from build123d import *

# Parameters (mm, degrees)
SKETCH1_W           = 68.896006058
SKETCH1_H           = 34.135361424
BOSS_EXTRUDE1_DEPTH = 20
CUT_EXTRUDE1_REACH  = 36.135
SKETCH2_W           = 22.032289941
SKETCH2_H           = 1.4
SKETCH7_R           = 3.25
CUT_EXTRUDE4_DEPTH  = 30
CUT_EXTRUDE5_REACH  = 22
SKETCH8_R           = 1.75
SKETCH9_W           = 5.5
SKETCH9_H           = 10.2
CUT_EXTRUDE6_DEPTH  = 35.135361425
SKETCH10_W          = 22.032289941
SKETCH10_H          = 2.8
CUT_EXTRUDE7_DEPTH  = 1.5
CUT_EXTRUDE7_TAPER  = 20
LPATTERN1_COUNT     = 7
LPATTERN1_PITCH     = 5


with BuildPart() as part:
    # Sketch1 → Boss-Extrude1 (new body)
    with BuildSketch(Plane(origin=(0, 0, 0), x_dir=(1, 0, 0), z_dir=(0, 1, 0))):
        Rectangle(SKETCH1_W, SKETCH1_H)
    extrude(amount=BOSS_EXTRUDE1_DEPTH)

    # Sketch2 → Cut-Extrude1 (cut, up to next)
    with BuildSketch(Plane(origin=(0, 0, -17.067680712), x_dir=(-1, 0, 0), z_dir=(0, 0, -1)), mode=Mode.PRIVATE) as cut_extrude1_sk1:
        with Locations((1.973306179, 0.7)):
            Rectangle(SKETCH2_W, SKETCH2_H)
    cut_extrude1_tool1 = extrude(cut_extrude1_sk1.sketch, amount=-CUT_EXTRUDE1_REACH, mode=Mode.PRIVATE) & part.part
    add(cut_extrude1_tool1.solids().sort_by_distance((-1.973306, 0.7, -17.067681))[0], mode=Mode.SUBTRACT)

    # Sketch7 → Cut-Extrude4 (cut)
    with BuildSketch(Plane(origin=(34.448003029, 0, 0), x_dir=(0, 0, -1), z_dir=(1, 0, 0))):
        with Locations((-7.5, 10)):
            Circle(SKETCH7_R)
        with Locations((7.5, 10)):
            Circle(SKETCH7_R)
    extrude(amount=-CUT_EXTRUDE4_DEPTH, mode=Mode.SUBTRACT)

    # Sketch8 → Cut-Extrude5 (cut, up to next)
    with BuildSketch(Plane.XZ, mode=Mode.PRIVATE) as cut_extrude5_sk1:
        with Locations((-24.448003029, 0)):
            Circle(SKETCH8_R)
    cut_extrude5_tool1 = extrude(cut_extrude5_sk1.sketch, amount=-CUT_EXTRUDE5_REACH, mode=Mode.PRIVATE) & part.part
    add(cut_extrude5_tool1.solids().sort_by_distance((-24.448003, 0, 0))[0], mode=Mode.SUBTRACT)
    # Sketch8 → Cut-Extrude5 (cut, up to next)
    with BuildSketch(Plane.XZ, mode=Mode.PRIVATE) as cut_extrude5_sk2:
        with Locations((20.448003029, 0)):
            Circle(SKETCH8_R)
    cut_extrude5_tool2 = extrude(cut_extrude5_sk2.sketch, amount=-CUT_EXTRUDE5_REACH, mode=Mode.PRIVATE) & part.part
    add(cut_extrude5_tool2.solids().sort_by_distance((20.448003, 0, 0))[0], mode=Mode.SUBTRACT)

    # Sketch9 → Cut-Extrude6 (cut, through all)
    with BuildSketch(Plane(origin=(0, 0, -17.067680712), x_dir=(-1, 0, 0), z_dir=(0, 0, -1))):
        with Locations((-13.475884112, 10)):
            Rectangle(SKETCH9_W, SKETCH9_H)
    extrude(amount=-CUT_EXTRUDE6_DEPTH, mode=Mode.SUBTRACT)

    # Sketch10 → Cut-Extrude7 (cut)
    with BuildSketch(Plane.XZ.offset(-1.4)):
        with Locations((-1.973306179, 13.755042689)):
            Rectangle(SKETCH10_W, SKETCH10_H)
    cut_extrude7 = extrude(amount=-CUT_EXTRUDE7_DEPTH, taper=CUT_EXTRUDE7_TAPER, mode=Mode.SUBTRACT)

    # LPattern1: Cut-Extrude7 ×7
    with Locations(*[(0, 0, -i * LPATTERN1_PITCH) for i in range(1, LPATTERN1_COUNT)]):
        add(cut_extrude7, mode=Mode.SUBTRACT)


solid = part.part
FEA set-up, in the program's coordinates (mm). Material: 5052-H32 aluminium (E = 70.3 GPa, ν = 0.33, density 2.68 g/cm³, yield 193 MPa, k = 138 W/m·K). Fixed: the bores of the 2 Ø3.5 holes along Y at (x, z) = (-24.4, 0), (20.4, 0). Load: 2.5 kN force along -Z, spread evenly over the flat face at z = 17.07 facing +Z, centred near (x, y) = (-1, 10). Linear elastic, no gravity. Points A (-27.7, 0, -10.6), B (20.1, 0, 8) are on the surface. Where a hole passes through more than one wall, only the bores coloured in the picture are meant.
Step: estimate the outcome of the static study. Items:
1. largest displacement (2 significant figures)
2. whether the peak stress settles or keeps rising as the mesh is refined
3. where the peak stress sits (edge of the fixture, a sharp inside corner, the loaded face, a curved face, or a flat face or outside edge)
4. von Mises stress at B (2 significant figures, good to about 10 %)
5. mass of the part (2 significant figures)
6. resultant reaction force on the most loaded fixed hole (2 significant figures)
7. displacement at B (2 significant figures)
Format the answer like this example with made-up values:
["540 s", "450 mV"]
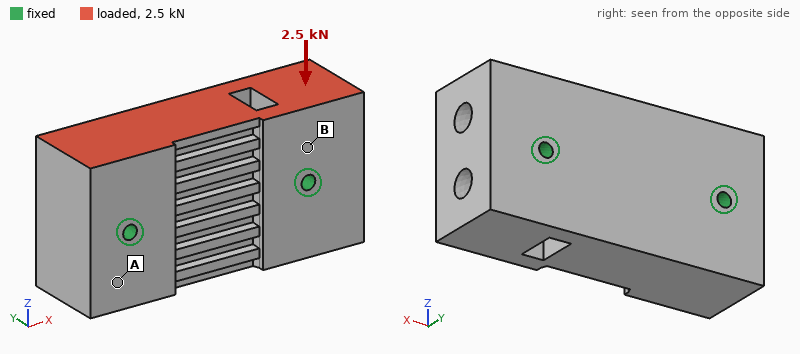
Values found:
["1.8 µm", "keeps rising", "edge of the fixture", "3.3 MPa", "110 g", "1.3 kN", "0.57 µm"]
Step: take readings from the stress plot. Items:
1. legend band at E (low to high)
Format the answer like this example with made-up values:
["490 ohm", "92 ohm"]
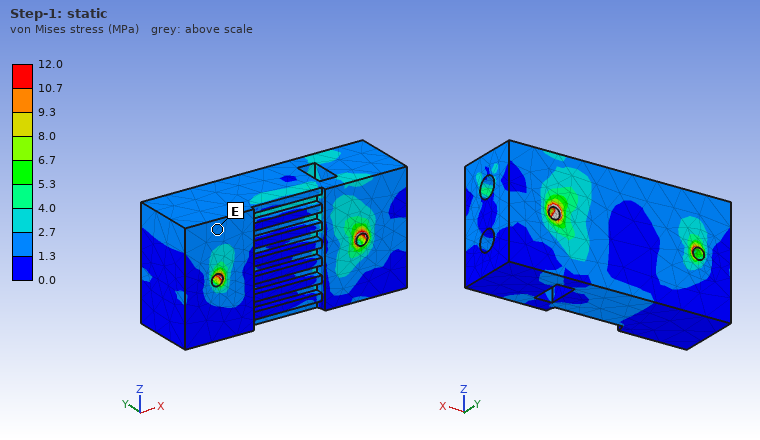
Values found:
["1.3 to 2.7 MPa"]
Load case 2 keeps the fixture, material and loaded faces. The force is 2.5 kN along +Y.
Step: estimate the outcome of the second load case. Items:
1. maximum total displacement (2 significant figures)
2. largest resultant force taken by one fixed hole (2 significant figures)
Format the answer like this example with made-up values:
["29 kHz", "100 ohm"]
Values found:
["9.6 µm", "1.3 kN"]
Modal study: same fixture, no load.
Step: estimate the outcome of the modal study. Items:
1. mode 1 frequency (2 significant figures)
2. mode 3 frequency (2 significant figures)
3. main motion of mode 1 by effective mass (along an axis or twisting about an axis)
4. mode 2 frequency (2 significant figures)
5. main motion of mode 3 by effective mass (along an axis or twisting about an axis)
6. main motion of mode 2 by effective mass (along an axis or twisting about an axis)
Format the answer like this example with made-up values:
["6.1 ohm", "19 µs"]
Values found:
["17 kHz", "21 kHz", "along Y", "18 kHz", "along Z", "twisting about X"]
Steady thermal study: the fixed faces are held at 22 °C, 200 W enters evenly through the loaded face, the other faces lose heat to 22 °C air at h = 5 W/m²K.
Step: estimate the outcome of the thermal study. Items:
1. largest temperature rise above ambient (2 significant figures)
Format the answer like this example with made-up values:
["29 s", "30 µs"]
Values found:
["34 K"]
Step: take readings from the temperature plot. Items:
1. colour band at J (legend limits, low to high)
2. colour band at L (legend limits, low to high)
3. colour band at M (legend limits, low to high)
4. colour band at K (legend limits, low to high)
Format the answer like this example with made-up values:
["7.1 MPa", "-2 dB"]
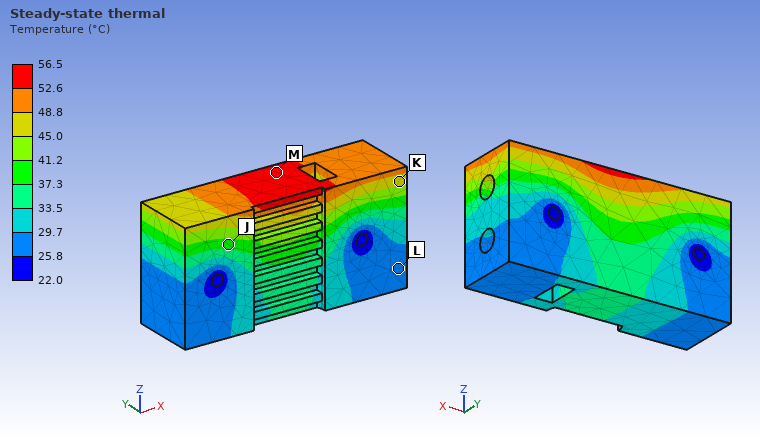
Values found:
["37.3 to 41.2 °C", "25.8 to 29.7 °C", "52.6 to 56.5 °C", "45.0 to 48.8 °C"]
